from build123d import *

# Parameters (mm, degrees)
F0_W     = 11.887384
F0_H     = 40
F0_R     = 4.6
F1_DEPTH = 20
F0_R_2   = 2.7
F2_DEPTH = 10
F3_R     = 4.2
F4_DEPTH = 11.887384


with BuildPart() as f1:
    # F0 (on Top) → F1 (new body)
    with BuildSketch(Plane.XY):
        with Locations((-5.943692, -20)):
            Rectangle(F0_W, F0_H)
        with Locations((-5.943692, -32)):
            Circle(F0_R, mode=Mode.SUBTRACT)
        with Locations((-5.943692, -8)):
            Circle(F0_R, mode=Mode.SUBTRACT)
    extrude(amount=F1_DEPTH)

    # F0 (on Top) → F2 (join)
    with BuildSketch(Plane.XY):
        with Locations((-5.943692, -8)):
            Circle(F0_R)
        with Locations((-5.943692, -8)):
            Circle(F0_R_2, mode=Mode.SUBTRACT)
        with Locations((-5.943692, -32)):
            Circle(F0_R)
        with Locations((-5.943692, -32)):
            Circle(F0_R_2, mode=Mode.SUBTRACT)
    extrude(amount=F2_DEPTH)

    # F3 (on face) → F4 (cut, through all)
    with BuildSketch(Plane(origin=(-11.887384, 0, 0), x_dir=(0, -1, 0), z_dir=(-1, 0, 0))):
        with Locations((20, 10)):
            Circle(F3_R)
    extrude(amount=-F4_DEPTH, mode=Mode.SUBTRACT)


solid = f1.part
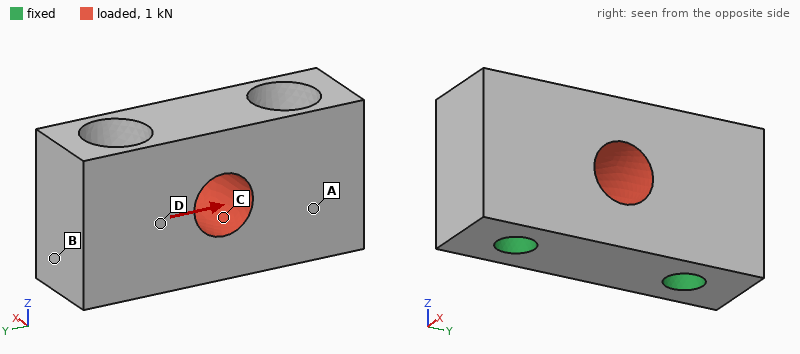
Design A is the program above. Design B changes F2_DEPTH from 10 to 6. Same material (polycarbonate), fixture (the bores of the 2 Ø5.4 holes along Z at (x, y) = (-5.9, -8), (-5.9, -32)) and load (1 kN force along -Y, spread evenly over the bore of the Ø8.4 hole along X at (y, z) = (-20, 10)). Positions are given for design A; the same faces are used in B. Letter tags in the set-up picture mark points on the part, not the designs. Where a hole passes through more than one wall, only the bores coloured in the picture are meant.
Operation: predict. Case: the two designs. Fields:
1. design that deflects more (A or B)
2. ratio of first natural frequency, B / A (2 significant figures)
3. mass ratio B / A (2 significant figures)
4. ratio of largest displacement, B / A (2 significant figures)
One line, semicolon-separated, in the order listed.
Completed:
B; 0.64; 0.95; 1.9
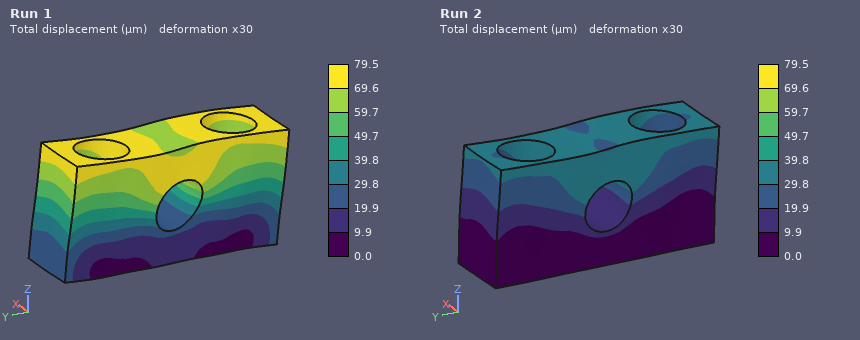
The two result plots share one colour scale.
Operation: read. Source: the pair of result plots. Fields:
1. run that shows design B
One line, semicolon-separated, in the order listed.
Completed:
Run 1
